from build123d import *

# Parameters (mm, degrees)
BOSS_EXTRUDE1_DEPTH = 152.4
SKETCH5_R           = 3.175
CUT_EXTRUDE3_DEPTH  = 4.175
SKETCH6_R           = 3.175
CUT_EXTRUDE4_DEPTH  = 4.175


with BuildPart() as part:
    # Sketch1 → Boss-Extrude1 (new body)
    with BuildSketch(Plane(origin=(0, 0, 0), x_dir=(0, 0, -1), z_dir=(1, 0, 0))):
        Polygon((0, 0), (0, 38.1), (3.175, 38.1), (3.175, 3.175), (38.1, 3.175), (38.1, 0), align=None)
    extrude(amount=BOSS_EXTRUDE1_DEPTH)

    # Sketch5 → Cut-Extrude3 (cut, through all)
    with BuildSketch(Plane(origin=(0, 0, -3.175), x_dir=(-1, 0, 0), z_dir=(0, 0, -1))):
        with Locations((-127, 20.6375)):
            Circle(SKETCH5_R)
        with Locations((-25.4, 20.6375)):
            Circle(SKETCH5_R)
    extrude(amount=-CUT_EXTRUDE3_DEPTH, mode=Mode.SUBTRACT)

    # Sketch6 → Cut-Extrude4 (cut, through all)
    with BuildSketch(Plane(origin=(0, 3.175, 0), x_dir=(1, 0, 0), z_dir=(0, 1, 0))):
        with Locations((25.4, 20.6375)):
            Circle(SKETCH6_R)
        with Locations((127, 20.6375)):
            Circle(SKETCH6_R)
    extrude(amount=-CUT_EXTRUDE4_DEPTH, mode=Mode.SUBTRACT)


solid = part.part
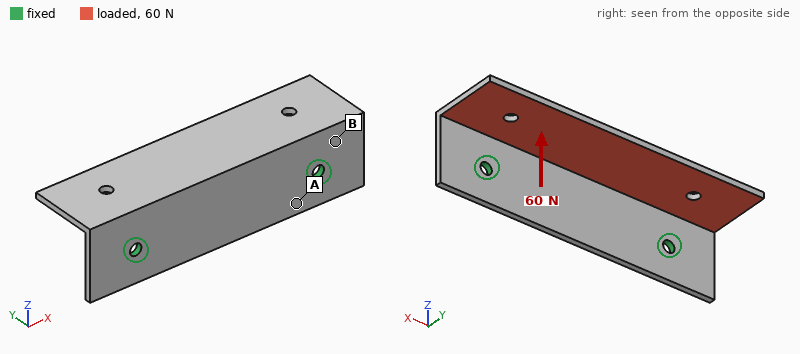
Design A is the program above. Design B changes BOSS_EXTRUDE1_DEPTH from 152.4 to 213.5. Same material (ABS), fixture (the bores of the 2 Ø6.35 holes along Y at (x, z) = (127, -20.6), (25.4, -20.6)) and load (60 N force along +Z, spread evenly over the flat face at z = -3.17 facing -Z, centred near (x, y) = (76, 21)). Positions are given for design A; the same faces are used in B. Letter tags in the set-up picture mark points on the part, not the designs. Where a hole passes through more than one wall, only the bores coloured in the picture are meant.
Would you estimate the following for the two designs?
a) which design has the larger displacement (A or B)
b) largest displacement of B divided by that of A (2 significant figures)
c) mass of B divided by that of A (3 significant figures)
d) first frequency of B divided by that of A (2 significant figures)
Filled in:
B
1.4
1.41
0.77
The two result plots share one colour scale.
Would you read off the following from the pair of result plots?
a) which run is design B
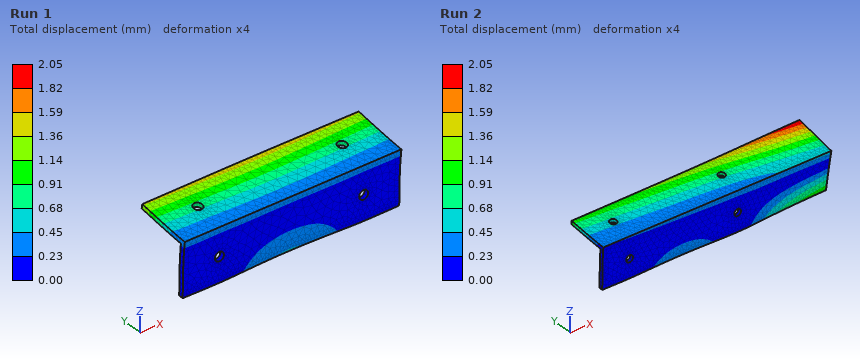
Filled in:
Run 2
